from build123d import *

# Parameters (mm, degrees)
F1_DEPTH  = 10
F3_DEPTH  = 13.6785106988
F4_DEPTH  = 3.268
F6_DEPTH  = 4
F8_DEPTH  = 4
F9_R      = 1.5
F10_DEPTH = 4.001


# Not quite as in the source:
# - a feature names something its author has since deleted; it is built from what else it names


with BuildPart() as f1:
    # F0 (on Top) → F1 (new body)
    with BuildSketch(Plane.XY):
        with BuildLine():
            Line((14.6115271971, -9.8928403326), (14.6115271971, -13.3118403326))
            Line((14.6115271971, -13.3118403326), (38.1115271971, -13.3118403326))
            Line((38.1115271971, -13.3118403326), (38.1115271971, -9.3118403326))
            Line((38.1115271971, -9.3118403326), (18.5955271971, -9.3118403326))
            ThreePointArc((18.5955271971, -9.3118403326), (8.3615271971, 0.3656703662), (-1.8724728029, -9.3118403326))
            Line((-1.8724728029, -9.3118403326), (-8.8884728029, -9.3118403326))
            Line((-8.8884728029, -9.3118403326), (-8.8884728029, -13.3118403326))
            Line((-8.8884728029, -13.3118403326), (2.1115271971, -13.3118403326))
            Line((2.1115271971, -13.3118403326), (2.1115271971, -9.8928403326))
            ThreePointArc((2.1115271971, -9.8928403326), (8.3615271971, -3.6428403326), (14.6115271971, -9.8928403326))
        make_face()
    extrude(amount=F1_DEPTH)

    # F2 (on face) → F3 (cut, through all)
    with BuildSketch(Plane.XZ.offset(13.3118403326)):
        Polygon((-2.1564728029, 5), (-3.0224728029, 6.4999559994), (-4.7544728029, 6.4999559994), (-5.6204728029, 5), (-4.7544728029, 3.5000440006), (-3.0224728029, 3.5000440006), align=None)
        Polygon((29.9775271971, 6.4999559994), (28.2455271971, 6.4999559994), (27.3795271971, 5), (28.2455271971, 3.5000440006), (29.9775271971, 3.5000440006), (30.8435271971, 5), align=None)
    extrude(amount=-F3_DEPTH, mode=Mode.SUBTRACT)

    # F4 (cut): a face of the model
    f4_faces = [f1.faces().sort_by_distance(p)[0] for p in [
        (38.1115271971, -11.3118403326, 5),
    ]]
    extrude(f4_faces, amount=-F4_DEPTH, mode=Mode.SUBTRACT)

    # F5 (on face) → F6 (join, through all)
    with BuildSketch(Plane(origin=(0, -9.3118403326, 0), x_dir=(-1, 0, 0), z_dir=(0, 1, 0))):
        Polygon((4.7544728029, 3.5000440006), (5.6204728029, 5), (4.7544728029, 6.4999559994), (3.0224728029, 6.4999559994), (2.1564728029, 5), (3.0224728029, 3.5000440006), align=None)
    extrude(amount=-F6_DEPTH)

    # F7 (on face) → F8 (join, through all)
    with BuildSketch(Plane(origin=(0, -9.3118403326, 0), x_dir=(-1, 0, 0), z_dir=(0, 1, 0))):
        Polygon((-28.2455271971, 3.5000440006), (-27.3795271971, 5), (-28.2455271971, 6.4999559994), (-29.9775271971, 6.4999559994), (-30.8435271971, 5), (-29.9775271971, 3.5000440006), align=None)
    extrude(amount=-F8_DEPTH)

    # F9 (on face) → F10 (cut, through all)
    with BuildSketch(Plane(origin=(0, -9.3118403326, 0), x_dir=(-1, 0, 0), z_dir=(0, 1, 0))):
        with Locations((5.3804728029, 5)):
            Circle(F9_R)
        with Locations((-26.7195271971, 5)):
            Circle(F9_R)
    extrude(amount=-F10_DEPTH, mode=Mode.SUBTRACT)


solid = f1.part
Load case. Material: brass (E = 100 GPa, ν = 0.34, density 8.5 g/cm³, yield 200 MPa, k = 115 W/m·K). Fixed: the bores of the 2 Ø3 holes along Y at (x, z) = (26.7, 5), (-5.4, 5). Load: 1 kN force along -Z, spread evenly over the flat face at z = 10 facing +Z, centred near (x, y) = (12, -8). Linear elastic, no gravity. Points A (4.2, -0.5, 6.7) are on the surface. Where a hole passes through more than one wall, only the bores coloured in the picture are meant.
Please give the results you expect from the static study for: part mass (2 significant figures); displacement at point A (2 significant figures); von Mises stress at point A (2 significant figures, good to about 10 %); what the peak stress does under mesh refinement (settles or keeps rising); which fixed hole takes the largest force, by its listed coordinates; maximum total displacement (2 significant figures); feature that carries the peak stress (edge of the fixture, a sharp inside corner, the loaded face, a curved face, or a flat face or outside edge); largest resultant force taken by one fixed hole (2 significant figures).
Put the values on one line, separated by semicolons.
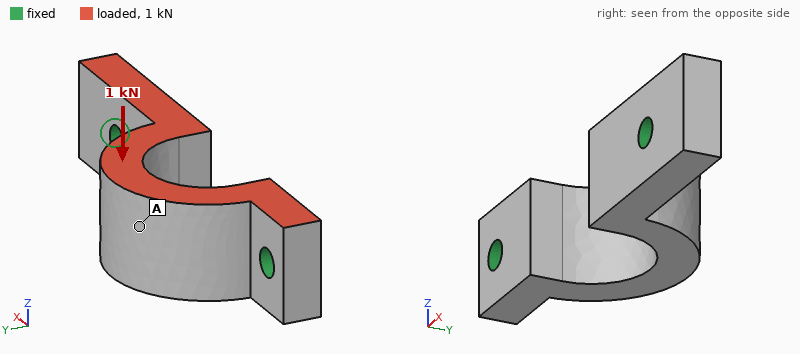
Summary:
19 g; 22 µm; 14 MPa; keeps rising; (26.7, 5); 27 µm; edge of the fixture; 530 N
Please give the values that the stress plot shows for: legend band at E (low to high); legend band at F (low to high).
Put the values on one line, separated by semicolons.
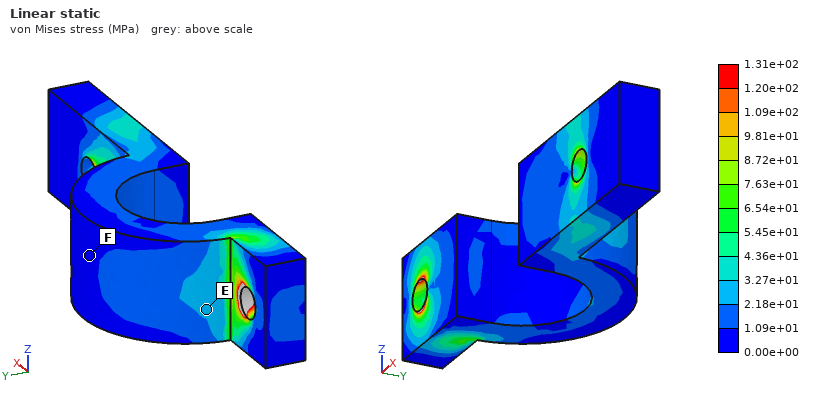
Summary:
2.18e+01 to 3.27e+01 MPa; 0.00e+00 to 1.09e+01 MPa
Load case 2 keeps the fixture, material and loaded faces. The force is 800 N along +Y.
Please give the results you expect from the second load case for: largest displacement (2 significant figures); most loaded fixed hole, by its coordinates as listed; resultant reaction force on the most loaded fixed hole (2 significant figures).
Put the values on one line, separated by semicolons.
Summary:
20 µm; (26.7, 5); 460 N
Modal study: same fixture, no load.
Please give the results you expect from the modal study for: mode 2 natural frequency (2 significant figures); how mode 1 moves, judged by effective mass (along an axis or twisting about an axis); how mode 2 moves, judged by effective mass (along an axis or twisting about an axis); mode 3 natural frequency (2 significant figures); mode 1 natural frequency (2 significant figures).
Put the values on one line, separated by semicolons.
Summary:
14 kHz; along Z; along Y; 20 kHz; 8400 Hz
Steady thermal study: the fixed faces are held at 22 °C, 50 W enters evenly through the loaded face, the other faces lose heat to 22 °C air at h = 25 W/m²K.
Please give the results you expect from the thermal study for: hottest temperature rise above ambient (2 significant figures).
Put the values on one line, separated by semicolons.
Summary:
49 K
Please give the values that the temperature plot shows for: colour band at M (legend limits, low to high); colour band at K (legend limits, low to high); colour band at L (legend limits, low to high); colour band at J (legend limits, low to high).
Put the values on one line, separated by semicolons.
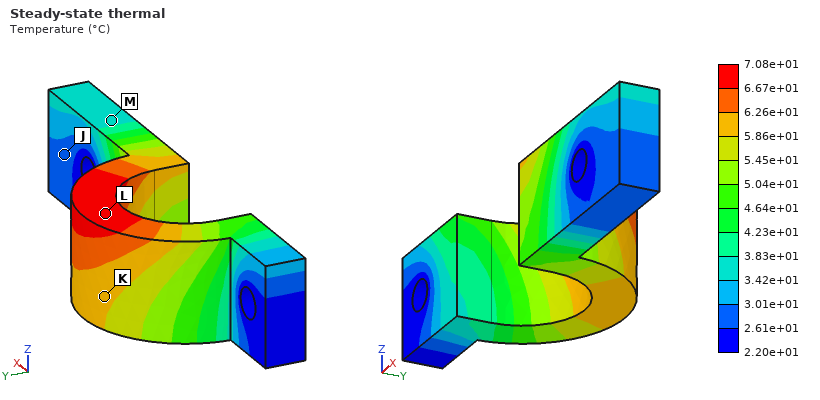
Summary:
3.42e+01 to 3.83e+01 °C; 5.86e+01 to 6.26e+01 °C; 6.67e+01 to 7.08e+01 °C; 2.61e+01 to 3.01e+01 °C
